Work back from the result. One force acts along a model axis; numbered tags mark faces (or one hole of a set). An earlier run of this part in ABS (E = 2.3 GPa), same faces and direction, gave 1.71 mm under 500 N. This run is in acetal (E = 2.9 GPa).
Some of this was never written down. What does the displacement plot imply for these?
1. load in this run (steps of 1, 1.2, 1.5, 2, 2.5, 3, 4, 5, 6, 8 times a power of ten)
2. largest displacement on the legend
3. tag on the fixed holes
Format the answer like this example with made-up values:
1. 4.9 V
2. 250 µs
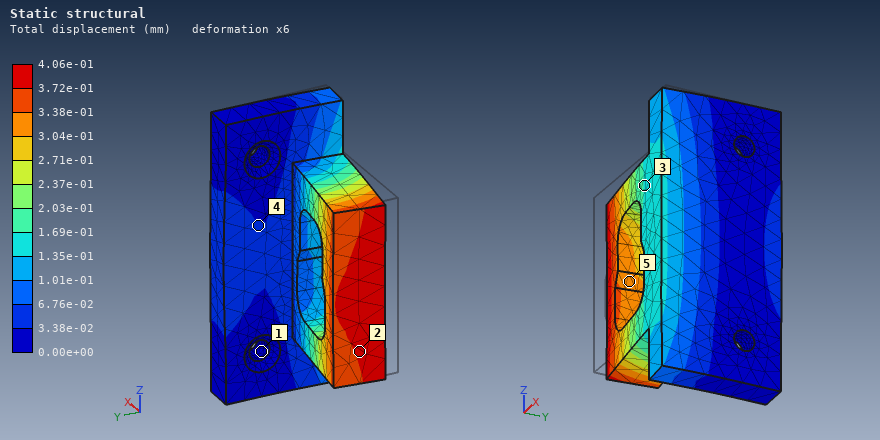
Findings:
1. 150 N
2. 4.06e-01 mm
3. 1
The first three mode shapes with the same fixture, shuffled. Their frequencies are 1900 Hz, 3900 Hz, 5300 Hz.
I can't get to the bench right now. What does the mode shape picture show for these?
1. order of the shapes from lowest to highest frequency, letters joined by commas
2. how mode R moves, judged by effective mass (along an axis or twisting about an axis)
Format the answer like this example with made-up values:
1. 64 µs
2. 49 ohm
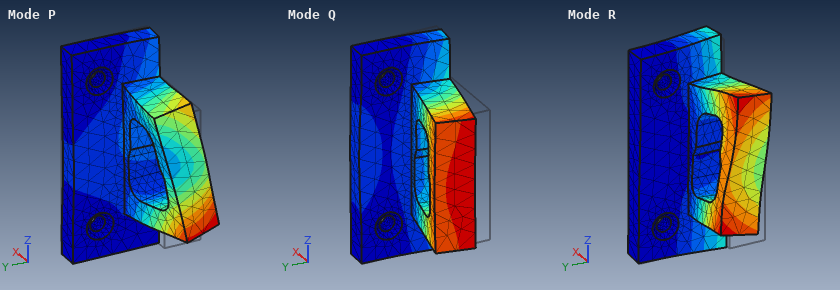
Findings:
1. Q, R, P
2. along Z
